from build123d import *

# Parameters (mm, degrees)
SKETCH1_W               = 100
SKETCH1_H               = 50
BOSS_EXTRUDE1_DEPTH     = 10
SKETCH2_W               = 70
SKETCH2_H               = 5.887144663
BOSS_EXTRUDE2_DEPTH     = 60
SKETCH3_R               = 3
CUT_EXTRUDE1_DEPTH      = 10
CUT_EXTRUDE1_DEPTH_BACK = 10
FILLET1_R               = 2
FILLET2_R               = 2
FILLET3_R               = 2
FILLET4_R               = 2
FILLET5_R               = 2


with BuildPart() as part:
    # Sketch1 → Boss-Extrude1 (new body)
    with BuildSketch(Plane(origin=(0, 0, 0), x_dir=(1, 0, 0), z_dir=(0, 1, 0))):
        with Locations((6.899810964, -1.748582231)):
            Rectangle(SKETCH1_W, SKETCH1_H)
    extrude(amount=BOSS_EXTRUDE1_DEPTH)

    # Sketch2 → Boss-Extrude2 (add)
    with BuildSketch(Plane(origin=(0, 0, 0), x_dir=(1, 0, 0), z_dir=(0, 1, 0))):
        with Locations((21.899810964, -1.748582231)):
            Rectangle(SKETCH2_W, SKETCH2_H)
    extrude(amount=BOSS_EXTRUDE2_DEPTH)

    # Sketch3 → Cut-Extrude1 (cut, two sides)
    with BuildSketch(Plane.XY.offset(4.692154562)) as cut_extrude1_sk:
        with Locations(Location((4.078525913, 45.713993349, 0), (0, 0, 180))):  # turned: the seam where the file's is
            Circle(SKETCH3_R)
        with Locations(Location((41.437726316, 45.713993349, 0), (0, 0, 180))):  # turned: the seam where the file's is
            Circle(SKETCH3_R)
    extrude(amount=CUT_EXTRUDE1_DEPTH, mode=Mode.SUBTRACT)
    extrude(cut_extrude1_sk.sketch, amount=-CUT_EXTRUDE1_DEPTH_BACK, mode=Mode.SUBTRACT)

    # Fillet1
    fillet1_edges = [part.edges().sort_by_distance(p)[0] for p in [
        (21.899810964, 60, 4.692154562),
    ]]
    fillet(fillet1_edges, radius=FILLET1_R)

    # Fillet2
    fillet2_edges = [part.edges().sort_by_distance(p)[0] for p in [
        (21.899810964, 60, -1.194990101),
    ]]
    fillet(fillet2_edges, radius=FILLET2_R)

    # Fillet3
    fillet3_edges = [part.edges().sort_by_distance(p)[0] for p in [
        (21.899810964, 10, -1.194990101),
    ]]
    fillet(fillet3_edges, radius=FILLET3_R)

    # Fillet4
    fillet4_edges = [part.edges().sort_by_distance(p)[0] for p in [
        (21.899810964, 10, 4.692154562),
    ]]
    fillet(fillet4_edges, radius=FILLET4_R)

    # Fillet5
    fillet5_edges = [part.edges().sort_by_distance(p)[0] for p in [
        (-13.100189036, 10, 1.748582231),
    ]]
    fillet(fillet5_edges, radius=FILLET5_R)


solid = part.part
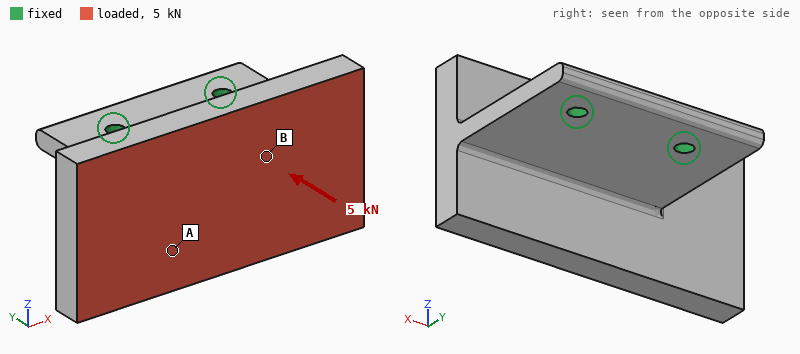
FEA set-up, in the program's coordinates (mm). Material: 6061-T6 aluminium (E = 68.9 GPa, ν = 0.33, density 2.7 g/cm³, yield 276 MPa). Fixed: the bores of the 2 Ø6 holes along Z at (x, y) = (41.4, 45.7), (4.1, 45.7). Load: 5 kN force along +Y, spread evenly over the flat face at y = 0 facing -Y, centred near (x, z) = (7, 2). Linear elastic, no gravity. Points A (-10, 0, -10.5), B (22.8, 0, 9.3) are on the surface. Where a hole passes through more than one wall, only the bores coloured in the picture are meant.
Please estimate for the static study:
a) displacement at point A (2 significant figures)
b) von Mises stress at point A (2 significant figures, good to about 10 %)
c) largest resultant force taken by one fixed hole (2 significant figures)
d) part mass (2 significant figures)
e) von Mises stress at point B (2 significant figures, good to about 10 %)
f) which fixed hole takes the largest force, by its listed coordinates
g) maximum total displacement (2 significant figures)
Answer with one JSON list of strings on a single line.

["33 µm", "22 MPa", "4.5 kN", "190 g", "8.3 MPa", "(4.1, 45.7)", "97 µm"]
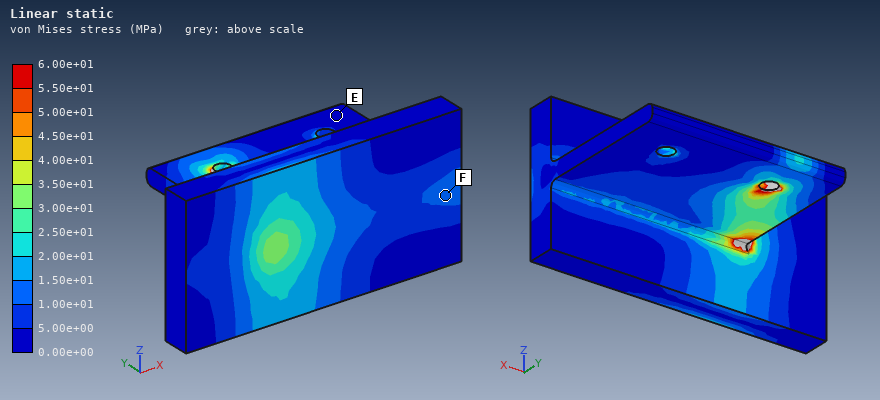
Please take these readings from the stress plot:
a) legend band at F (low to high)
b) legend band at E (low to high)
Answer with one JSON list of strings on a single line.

["1.00e+01 to 1.50e+01 MPa", "0.00e+00 to 5.00e+00 MPa"]
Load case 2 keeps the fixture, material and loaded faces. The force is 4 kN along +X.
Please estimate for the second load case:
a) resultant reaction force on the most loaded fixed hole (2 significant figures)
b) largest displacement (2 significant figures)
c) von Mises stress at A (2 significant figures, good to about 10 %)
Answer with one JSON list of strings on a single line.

["4.9 kN", "76 µm", "9.4 MPa"]
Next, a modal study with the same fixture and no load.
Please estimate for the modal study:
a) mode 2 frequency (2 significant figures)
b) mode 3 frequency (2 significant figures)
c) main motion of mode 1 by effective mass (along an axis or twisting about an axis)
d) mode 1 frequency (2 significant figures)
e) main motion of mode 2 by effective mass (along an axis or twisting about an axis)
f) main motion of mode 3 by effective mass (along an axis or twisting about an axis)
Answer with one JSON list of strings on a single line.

["1300 Hz", "3300 Hz", "along Z", "680 Hz", "twisting about Y", "along Z"]
